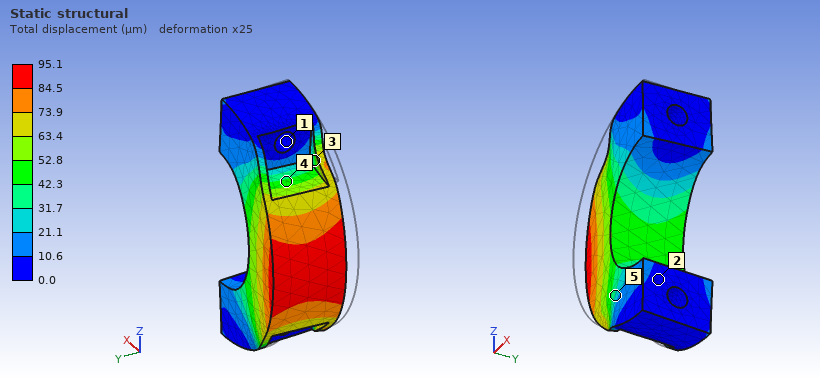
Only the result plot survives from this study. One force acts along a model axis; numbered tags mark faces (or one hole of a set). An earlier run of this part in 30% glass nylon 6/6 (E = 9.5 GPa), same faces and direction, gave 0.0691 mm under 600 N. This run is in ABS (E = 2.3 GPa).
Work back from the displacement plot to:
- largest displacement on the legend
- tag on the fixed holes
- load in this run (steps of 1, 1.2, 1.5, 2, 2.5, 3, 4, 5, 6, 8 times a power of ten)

95.1 µm
1
200 N
